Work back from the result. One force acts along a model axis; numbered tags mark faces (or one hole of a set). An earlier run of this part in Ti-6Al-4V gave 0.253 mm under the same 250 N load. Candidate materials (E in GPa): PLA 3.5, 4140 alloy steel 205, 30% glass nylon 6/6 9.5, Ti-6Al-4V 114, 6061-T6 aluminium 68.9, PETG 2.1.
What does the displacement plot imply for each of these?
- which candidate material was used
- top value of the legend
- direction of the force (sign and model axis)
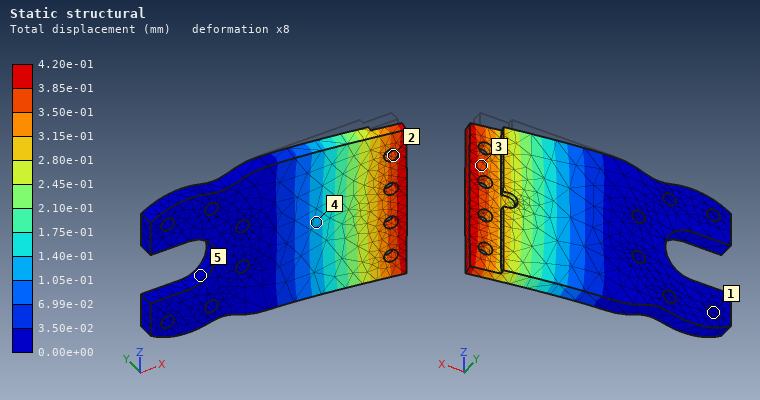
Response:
6061-T6 aluminium
4.20e-01 mm
-Y
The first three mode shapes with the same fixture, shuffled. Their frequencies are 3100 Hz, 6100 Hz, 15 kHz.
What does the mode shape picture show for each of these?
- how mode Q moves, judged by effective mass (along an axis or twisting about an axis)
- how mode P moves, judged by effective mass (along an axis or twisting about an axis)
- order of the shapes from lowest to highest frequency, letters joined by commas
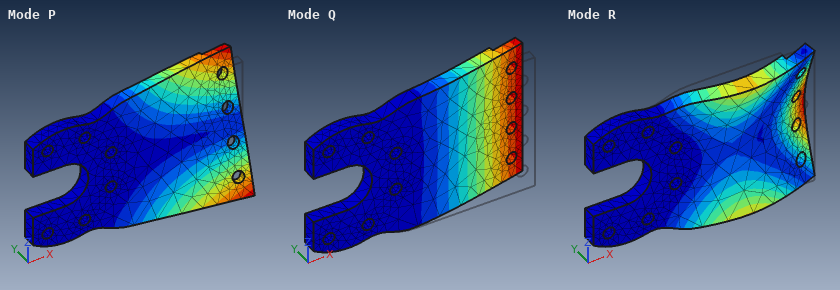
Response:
along Y
twisting about X
Q, P, R
